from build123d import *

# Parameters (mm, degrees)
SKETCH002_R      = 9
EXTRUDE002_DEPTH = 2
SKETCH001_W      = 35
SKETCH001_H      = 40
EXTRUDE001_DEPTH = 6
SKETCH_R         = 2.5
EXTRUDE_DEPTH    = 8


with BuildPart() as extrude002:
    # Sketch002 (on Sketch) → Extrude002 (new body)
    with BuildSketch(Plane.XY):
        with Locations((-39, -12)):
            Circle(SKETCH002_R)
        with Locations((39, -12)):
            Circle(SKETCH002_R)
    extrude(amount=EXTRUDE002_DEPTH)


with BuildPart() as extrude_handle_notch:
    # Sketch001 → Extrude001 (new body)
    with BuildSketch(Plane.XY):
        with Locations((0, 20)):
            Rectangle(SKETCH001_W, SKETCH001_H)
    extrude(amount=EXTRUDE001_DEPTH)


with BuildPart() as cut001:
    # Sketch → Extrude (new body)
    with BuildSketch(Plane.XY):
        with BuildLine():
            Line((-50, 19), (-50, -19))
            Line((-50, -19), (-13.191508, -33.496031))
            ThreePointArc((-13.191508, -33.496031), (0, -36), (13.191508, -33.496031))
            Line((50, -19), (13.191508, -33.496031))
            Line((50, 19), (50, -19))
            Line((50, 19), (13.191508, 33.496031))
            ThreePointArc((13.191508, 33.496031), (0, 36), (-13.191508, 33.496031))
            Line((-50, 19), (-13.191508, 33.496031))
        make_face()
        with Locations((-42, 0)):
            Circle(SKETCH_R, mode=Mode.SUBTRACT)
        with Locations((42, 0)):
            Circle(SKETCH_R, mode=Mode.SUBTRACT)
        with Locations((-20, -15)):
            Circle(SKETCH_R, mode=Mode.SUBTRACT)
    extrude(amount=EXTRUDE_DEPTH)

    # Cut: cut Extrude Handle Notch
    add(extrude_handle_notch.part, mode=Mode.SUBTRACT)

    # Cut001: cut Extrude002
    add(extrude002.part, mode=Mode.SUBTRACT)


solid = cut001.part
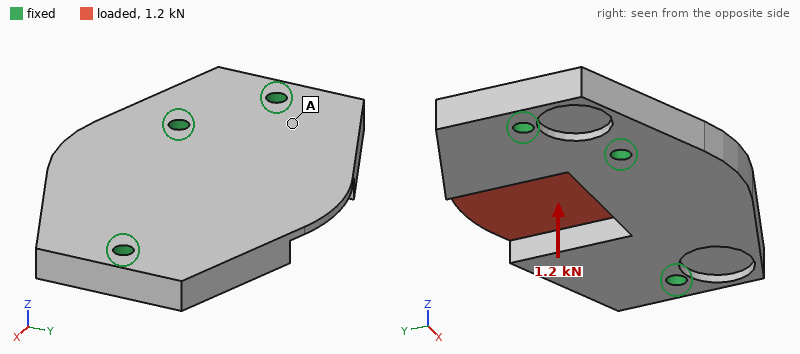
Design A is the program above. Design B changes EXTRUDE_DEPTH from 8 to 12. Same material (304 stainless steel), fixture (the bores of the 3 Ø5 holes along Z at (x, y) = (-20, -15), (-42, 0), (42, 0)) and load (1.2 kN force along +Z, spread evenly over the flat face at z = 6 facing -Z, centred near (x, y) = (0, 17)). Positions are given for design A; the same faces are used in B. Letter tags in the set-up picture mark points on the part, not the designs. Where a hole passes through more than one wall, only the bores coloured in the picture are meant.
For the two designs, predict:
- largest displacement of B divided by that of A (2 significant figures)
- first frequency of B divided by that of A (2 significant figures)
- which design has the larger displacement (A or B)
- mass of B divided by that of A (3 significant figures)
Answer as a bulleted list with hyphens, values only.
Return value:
- 0.18
- 1.3
- A
- 1.61
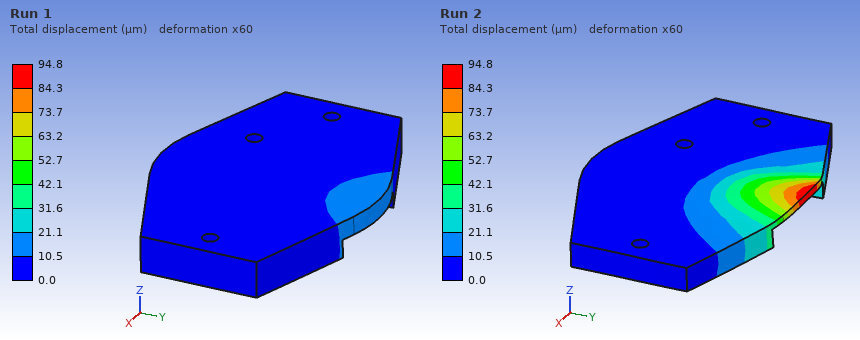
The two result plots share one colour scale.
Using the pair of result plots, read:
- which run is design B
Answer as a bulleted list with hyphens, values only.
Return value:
- Run 1
